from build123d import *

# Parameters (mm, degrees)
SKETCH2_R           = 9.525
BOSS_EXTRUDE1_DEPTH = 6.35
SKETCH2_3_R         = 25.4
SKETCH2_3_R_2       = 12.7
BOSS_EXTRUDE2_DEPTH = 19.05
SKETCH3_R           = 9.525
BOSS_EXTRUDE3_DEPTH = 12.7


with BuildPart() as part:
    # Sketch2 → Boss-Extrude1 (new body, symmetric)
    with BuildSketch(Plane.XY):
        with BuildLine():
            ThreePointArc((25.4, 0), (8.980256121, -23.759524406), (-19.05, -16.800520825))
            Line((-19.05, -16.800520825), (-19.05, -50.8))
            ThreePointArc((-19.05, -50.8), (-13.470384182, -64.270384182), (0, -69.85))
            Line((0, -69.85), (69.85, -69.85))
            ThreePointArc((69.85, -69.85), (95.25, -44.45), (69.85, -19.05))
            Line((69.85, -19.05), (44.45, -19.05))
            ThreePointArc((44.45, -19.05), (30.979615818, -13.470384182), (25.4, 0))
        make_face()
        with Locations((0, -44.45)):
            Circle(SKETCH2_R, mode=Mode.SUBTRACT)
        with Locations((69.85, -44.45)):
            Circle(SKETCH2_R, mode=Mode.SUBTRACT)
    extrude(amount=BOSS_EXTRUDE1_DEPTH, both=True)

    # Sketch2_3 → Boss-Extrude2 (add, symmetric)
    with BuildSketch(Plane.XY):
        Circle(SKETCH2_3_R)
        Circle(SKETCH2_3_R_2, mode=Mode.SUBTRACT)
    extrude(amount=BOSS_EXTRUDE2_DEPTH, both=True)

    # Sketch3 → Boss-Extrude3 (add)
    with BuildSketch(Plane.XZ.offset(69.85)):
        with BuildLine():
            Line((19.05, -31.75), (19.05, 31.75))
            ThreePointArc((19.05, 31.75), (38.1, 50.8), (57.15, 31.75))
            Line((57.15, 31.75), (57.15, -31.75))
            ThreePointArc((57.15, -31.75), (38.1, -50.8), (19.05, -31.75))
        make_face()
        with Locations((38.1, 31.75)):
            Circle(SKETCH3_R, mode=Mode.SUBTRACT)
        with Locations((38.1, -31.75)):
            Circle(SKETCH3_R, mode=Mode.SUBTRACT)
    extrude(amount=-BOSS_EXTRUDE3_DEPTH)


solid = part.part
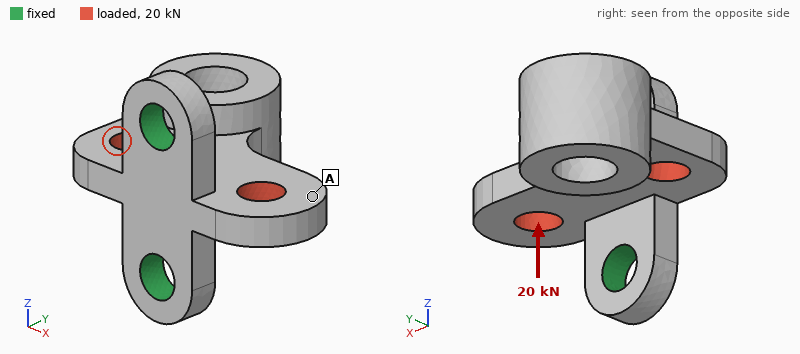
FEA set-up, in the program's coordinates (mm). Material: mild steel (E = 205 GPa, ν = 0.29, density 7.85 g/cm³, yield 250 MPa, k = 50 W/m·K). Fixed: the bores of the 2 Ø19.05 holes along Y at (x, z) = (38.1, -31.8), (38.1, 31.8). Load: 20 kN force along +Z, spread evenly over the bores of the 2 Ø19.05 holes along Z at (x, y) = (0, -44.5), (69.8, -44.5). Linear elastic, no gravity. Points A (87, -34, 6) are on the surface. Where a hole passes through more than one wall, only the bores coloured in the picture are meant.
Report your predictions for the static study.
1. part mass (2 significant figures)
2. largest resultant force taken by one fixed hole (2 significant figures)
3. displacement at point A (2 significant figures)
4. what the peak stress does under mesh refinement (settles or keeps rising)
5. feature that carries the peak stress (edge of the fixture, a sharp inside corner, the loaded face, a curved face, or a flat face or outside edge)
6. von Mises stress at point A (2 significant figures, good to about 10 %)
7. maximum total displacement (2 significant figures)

1.2 kg
14 kN
0.11 mm
keeps rising
a sharp inside corner
25 MPa
0.26 mm
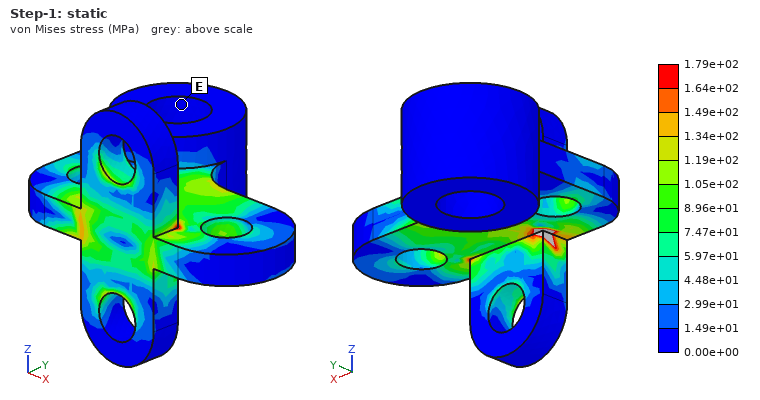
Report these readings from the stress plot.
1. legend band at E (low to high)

0.00e+00 to 1.49e+01 MPa
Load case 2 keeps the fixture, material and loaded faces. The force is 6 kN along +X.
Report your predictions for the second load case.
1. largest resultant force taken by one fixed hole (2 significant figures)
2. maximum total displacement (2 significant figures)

3.0 kN
60 µm
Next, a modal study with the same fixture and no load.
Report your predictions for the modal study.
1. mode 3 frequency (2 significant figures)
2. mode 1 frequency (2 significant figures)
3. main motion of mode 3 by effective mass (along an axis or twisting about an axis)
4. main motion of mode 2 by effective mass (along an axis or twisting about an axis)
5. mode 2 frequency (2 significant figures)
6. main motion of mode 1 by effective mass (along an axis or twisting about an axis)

2700 Hz
840 Hz
twisting about Y
along X
1200 Hz
along Z
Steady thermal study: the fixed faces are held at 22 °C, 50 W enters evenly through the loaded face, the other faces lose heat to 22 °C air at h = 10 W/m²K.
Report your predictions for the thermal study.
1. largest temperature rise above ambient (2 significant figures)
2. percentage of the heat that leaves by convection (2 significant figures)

51 K
18 %
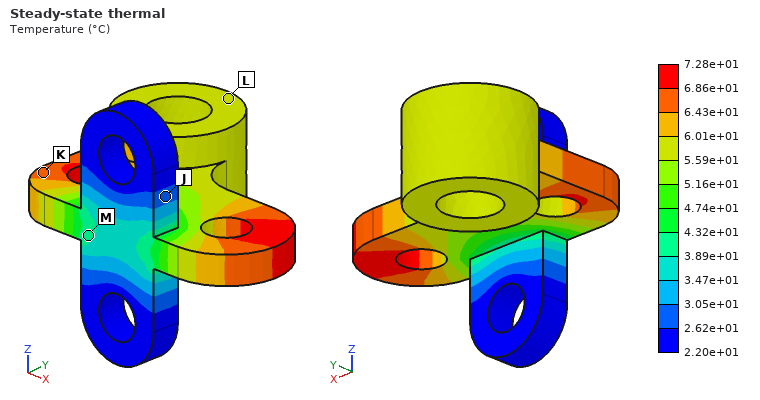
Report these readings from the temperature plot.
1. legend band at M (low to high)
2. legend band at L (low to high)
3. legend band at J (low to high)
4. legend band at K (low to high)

3.89e+01 to 4.32e+01 °C
5.59e+01 to 6.01e+01 °C
2.62e+01 to 3.05e+01 °C
6.43e+01 to 6.86e+01 °C
